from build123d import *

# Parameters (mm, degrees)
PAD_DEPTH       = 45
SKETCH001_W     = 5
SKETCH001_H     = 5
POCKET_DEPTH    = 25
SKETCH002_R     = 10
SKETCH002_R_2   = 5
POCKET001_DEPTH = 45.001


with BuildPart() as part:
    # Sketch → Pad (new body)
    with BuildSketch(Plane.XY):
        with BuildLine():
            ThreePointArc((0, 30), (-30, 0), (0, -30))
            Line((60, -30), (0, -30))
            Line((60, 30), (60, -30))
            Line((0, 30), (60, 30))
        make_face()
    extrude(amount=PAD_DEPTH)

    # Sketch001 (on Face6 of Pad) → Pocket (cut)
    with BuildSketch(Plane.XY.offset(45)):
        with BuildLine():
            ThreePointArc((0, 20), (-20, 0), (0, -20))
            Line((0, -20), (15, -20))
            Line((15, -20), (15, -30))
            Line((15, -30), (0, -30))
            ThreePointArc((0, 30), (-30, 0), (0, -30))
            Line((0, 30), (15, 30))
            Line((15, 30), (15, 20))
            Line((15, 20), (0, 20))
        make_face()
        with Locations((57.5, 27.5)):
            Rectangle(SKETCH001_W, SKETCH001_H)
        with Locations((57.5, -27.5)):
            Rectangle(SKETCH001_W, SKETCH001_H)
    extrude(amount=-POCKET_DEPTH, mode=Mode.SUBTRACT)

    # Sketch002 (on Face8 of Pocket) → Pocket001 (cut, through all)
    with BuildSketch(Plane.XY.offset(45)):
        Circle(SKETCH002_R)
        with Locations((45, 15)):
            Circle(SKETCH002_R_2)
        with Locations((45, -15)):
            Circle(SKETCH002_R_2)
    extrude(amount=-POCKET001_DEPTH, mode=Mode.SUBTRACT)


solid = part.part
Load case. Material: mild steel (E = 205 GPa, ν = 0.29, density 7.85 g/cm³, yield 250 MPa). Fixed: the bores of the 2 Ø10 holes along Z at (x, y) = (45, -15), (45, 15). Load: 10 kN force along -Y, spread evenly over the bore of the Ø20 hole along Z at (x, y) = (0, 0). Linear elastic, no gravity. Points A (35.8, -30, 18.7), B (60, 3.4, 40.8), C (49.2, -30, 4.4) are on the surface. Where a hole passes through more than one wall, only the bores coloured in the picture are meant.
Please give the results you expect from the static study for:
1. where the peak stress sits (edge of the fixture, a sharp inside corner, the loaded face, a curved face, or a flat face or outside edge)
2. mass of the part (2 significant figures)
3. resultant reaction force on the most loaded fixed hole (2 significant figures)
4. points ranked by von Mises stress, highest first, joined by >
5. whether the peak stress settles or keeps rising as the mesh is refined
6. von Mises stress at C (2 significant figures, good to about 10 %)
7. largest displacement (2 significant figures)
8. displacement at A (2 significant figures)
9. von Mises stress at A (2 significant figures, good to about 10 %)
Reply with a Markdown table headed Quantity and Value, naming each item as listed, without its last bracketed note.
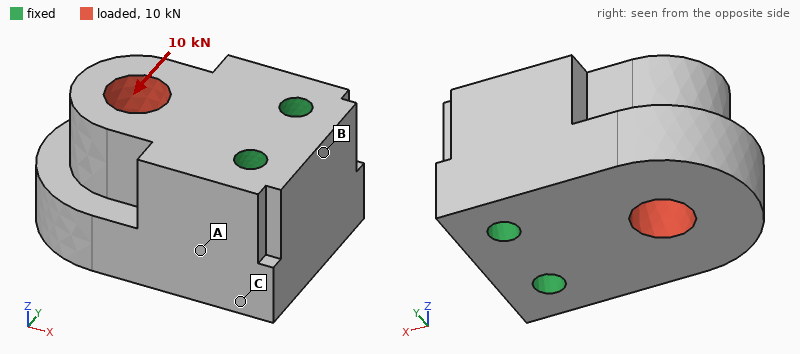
| Quantity | Value |
|---|---|
| where the peak stress sits | edge of the fixture |
| mass of the part | 1.4 kg |
| resultant reaction force on the most loaded fixed hole | 13 kN |
| points ranked by von Mises stress, highest first, joined by > | A > C > B |
| whether the peak stress settles or keeps rising as the mesh is refined | keeps rising |
| von Mises stress at C | 5.7 MPa |
| largest displacement | 9.0 µm |
| displacement at A | 1.7 µm |
| von Mises stress at A | 9.9 MPa |
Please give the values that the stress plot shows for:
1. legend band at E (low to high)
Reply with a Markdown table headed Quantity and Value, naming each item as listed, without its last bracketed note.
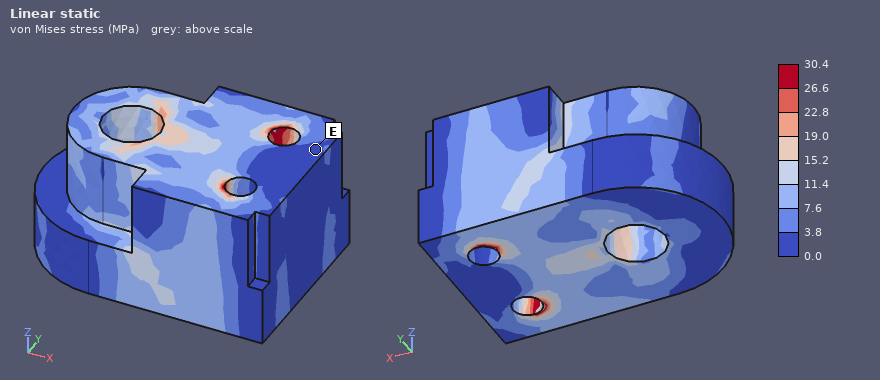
| Quantity | Value |
|---|---|
| legend band at E | 0.0 to 3.8 MPa |
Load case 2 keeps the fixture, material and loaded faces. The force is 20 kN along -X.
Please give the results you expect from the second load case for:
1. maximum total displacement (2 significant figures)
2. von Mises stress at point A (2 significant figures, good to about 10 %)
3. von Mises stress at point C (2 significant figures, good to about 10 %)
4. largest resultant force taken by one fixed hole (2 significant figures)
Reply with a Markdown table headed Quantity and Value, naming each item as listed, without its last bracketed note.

| Quantity | Value |
|---|---|
| maximum total displacement | 4.3 µm |
| von Mises stress at point A | 3.6 MPa |
| von Mises stress at point C | 2.7 MPa |
| largest resultant force taken by one fixed hole | 10 kN |
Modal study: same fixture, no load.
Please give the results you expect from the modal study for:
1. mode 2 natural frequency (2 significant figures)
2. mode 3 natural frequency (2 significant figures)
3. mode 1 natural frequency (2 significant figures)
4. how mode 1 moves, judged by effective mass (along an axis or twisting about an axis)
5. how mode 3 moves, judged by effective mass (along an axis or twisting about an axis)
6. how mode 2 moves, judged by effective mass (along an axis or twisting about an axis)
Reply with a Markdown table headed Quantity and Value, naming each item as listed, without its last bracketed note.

| Quantity | Value |
|---|---|
| mode 2 natural frequency | 7600 Hz |
| mode 3 natural frequency | 12 kHz |
| mode 1 natural frequency | 7100 Hz |
| how mode 1 moves, judged by effective mass | along Z |
| how mode 3 moves, judged by effective mass | twisting about X |
| how mode 2 moves, judged by effective mass | along Y |
